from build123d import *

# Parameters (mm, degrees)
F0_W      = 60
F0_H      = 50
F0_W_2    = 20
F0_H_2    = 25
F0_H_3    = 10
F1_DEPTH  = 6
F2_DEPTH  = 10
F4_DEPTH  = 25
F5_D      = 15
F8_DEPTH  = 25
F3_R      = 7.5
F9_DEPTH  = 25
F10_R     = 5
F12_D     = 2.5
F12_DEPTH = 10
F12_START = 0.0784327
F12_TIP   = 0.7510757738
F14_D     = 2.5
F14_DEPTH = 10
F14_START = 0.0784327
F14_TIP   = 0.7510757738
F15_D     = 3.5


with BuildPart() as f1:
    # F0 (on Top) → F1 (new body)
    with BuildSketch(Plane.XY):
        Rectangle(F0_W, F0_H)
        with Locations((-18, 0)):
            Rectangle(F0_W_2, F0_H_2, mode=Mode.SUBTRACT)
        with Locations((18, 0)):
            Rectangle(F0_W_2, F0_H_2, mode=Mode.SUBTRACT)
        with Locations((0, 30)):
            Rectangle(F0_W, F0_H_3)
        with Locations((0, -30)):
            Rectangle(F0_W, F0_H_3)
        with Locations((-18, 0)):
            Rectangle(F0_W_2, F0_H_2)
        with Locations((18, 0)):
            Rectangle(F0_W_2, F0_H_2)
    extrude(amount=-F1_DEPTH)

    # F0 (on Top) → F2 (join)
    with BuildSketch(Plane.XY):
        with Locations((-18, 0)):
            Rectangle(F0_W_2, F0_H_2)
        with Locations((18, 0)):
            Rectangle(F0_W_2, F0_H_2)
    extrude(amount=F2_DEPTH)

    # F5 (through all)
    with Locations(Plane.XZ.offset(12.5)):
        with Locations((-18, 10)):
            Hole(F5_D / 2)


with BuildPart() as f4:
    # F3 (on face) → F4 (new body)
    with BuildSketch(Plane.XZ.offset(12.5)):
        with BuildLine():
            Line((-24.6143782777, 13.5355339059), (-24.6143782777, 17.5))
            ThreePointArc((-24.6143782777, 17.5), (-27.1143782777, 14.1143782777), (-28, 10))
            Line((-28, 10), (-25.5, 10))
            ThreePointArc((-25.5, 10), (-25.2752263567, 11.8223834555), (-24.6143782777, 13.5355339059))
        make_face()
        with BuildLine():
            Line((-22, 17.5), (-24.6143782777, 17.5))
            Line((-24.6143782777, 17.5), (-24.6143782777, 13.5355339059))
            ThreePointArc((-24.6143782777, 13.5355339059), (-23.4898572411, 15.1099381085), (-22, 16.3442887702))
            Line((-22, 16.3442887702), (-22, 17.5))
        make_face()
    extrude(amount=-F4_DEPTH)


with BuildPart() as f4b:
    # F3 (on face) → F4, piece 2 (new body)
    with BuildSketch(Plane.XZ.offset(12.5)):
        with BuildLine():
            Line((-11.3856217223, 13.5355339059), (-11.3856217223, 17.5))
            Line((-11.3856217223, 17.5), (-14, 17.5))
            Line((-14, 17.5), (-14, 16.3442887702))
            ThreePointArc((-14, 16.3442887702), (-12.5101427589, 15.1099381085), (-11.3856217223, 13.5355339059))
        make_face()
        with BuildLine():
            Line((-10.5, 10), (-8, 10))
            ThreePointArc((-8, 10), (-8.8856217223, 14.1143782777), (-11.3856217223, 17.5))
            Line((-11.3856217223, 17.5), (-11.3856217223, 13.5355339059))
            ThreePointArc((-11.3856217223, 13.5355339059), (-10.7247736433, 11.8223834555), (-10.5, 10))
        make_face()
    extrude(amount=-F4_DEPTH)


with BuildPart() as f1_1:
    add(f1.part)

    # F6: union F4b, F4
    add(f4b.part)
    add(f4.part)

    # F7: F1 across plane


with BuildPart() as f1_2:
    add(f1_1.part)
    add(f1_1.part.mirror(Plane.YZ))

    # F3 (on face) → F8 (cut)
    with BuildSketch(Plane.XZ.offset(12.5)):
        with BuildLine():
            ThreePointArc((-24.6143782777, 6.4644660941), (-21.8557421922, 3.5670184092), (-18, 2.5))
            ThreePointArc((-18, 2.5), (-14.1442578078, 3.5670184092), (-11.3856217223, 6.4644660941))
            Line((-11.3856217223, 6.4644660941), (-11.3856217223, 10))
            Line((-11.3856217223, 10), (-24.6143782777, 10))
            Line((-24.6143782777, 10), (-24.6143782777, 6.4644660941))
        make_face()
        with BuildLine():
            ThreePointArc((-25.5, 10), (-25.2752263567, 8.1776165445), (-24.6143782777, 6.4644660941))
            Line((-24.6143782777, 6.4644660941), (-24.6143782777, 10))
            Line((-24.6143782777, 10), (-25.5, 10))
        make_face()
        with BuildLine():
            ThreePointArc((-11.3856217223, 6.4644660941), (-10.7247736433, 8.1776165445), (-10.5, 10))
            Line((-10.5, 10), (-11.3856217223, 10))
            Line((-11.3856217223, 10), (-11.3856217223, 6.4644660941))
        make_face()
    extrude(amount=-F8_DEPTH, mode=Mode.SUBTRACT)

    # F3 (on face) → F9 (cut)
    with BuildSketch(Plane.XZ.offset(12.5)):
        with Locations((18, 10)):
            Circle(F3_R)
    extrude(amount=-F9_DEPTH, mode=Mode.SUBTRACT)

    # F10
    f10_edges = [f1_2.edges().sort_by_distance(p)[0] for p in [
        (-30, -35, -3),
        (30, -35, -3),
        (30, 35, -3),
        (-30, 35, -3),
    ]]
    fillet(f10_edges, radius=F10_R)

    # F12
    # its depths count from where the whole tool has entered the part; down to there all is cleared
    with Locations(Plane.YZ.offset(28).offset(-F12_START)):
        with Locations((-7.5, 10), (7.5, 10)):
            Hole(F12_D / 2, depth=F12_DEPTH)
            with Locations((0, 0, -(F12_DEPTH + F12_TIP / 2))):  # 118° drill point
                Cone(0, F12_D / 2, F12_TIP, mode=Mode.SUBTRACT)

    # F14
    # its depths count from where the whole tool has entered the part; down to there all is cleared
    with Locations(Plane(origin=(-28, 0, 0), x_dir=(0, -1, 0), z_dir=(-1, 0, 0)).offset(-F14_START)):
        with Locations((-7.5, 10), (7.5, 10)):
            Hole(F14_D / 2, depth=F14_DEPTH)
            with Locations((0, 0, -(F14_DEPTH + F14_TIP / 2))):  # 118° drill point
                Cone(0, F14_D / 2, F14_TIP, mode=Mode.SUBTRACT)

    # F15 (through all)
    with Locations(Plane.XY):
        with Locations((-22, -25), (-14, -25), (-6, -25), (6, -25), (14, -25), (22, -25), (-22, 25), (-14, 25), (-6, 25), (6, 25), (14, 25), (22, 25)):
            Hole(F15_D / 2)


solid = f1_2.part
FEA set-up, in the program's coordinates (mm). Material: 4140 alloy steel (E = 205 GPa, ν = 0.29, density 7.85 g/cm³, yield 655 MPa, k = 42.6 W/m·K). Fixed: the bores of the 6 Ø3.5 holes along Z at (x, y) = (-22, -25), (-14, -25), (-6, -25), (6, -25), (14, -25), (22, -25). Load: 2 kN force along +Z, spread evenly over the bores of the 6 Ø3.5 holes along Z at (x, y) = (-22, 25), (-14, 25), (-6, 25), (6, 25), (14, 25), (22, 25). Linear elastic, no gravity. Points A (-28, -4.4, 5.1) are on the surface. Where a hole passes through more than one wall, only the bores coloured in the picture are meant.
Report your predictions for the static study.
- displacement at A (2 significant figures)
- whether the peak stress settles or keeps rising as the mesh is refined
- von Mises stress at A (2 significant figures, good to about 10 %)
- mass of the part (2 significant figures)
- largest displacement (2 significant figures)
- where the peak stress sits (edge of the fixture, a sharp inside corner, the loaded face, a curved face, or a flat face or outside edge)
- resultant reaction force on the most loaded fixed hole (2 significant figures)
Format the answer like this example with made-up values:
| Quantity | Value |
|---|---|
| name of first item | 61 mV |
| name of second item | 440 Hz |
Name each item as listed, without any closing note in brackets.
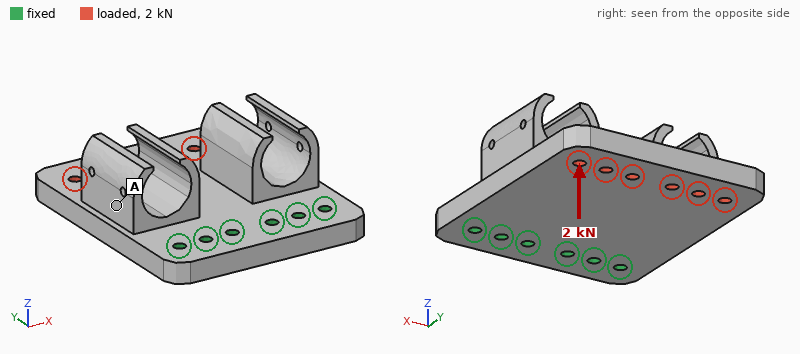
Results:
| Quantity | Value |
|---|---|
| displacement at A | 0.086 mm |
| whether the peak stress settles or keeps rising as the mesh is refined | keeps rising |
| von Mises stress at A | 32 MPa |
| mass of the part | 250 g |
| largest displacement | 0.34 mm |
| where the peak stress sits | edge of the fixture |
| resultant reaction force on the most loaded fixed hole | 550 N |
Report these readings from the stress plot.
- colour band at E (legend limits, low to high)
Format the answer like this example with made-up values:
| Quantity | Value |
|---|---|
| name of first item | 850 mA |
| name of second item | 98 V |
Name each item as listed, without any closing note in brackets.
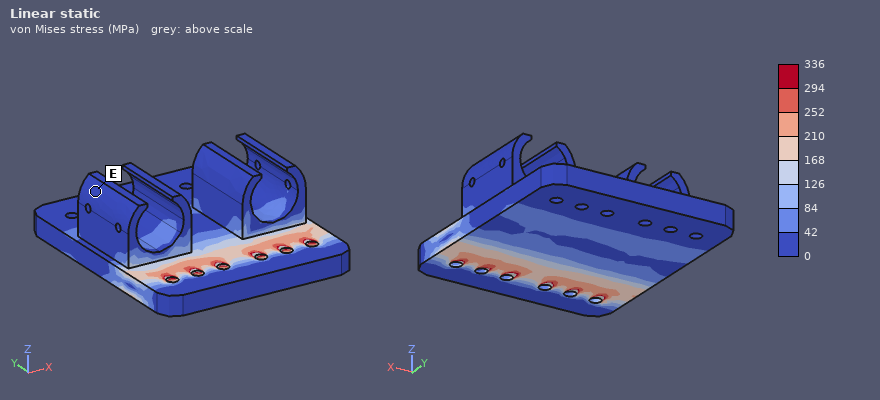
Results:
| Quantity | Value |
|---|---|
| colour band at E | 0 to 42 MPa |
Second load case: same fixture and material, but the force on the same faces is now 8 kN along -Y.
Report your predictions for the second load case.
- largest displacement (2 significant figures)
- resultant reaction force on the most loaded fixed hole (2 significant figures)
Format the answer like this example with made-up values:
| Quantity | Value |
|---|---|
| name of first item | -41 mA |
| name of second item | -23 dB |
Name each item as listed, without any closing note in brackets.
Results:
| Quantity | Value |
|---|---|
| largest displacement | 11 µm |
| resultant reaction force on the most loaded fixed hole | 1.7 kN |
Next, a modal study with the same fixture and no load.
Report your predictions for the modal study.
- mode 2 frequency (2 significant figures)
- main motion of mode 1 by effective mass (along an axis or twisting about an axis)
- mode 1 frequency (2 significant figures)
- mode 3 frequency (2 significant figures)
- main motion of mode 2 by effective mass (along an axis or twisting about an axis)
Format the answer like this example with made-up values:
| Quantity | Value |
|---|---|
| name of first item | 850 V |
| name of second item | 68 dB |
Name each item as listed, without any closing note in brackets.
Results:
| Quantity | Value |
|---|---|
| mode 2 frequency | 3500 Hz |
| main motion of mode 1 by effective mass | along Z |
| mode 1 frequency | 1500 Hz |
| mode 3 frequency | 7800 Hz |
| main motion of mode 2 by effective mass | twisting about Y |
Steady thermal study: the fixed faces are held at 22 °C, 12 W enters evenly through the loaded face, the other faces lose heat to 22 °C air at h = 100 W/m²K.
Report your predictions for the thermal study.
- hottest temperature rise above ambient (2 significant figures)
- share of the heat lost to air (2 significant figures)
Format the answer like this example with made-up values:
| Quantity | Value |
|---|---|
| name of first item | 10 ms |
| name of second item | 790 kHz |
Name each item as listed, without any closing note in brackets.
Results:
| Quantity | Value |
|---|---|
| hottest temperature rise above ambient | 18 K |
| share of the heat lost to air | 70 % |
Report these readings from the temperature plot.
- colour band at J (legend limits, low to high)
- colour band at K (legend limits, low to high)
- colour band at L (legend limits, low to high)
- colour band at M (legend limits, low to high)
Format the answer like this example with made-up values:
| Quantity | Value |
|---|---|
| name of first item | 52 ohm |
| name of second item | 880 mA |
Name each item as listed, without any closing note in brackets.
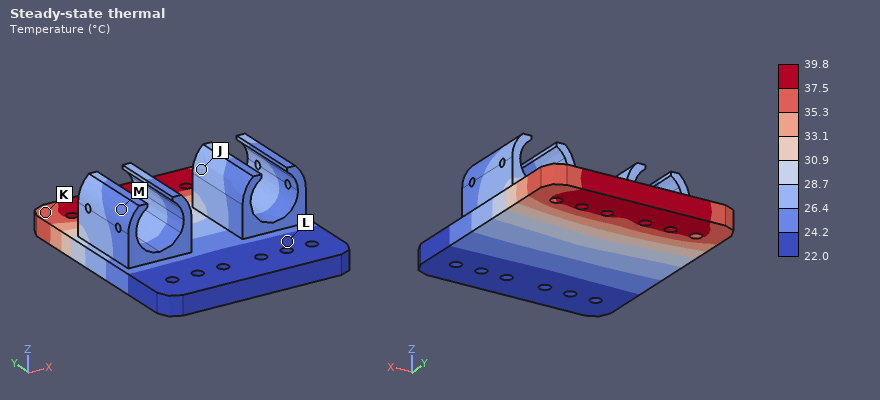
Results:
| Quantity | Value |
|---|---|
| colour band at J | 26.4 to 28.7 °C |
| colour band at K | 35.3 to 37.5 °C |
| colour band at L | 22.0 to 24.2 °C |
| colour band at M | 24.2 to 26.4 °C |
